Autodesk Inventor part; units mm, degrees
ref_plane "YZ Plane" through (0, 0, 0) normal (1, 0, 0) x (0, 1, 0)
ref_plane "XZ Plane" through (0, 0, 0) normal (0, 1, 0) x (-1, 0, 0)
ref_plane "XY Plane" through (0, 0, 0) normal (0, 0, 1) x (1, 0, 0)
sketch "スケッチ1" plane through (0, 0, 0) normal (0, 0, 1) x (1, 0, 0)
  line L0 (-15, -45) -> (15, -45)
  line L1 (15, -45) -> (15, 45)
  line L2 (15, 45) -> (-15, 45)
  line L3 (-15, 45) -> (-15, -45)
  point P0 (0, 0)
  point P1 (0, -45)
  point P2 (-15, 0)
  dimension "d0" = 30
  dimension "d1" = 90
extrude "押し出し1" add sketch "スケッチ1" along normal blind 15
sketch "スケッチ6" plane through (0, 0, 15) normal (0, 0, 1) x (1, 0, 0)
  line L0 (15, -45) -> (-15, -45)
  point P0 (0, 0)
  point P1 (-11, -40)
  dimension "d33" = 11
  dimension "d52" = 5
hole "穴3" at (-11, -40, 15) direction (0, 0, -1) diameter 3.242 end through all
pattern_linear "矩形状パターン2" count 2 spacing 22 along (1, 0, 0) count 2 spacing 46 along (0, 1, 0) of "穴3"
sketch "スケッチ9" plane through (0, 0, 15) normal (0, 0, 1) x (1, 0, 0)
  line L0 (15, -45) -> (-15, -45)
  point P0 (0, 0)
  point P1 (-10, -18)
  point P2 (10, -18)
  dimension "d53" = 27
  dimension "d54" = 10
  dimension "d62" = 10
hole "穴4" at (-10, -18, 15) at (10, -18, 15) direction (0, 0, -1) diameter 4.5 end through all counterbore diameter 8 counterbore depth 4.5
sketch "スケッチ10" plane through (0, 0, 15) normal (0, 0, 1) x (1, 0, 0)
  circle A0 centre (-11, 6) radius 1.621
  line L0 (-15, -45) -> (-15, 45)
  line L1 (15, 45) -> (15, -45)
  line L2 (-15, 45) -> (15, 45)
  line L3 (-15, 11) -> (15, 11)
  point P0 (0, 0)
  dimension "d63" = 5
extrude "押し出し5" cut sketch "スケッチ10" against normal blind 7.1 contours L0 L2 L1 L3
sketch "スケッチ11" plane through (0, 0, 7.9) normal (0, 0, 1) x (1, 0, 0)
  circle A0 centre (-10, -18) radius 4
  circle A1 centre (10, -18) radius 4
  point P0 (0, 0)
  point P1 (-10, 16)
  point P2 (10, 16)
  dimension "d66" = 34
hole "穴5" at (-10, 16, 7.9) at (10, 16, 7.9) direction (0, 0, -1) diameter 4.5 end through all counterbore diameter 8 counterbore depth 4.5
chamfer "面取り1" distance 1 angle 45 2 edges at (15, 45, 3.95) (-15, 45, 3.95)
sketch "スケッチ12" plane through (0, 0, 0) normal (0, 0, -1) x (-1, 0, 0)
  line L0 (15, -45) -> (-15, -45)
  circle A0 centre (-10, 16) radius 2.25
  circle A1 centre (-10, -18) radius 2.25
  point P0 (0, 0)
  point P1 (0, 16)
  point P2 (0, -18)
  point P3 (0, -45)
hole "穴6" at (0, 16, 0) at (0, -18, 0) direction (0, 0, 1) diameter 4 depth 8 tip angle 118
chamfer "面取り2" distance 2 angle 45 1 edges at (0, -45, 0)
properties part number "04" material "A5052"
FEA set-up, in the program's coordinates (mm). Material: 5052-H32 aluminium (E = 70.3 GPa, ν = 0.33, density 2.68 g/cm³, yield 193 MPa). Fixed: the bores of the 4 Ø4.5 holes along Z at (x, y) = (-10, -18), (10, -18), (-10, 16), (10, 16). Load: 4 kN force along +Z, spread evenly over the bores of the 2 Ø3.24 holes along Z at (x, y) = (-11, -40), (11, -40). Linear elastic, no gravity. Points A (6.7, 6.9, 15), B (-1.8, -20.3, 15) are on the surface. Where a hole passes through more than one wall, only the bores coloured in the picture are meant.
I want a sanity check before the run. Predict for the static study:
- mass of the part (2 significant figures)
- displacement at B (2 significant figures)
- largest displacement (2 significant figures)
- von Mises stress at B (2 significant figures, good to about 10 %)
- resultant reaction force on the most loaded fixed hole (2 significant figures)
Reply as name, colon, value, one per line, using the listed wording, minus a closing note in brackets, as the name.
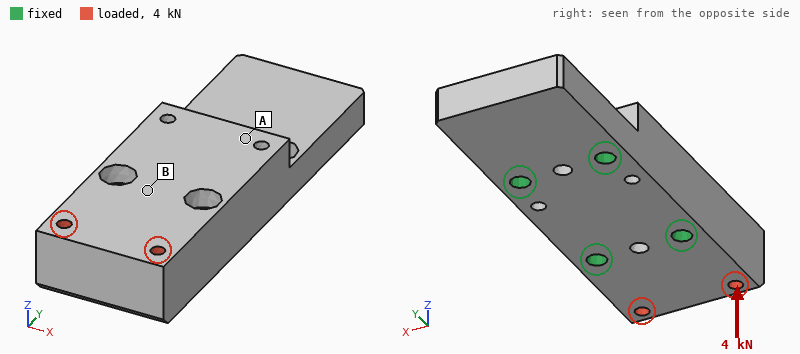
mass of the part: 83 g
displacement at B: 13 µm
largest displacement: 66 µm
von Mises stress at B: 59 MPa
resultant reaction force on the most loaded fixed hole: 2.5 kN
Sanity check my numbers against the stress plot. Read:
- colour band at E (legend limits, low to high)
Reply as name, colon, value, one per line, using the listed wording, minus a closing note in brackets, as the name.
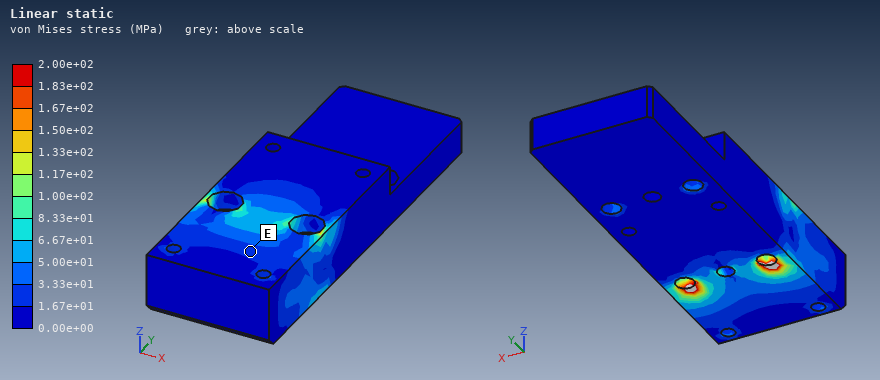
colour band at E: 1.67e+01 to 3.33e+01 MPa
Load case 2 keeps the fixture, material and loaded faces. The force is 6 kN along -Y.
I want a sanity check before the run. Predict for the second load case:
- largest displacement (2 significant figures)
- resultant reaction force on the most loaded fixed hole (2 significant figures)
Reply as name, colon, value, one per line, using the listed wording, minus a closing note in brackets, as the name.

largest displacement: 10 µm
resultant reaction force on the most loaded fixed hole: 2.8 kN
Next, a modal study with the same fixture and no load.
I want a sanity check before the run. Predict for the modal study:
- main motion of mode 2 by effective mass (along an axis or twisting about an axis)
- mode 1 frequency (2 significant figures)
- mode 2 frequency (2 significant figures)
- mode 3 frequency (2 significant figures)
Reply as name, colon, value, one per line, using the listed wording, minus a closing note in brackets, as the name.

main motion of mode 2 by effective mass: along Z
mode 1 frequency: 5500 Hz
mode 2 frequency: 11 kHz
mode 3 frequency: 13 kHz
